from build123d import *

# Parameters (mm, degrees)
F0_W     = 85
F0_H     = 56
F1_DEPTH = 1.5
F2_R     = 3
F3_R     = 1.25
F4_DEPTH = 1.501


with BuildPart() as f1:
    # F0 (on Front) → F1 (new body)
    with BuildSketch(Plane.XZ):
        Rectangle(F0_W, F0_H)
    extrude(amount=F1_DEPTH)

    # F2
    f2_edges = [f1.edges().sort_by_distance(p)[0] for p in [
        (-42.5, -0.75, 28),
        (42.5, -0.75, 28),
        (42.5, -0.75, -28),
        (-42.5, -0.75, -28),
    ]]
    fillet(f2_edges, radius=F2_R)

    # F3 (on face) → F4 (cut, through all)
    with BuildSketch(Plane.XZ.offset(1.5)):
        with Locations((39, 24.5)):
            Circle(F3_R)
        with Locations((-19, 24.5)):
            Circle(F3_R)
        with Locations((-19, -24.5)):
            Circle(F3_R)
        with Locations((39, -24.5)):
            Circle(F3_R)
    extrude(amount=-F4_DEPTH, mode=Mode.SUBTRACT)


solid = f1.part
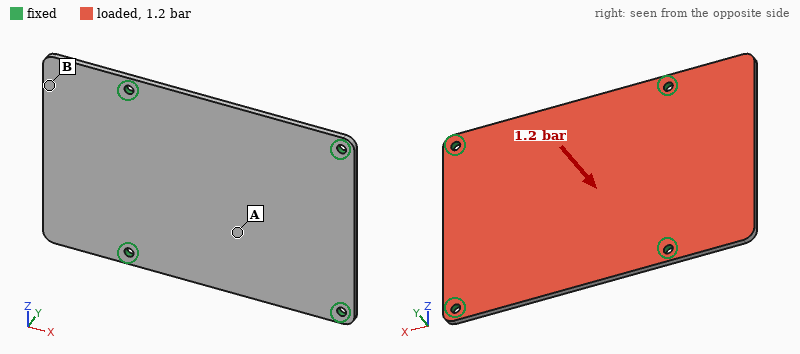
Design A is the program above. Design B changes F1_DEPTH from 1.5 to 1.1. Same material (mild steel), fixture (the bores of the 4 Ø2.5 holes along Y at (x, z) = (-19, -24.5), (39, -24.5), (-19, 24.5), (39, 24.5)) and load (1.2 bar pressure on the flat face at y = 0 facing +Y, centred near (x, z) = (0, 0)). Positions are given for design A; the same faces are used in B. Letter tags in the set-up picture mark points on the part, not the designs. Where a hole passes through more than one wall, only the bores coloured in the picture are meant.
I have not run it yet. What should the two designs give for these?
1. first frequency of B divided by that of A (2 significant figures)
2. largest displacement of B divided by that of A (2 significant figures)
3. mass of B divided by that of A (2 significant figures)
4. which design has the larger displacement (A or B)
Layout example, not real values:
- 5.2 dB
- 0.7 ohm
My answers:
- 0.74
- 2.5
- 0.73
- B
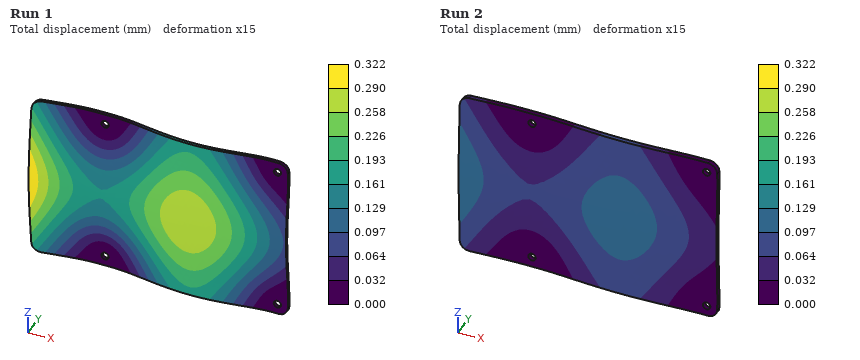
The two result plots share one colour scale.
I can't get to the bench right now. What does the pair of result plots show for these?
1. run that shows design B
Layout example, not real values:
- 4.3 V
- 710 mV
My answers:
- Run 1
